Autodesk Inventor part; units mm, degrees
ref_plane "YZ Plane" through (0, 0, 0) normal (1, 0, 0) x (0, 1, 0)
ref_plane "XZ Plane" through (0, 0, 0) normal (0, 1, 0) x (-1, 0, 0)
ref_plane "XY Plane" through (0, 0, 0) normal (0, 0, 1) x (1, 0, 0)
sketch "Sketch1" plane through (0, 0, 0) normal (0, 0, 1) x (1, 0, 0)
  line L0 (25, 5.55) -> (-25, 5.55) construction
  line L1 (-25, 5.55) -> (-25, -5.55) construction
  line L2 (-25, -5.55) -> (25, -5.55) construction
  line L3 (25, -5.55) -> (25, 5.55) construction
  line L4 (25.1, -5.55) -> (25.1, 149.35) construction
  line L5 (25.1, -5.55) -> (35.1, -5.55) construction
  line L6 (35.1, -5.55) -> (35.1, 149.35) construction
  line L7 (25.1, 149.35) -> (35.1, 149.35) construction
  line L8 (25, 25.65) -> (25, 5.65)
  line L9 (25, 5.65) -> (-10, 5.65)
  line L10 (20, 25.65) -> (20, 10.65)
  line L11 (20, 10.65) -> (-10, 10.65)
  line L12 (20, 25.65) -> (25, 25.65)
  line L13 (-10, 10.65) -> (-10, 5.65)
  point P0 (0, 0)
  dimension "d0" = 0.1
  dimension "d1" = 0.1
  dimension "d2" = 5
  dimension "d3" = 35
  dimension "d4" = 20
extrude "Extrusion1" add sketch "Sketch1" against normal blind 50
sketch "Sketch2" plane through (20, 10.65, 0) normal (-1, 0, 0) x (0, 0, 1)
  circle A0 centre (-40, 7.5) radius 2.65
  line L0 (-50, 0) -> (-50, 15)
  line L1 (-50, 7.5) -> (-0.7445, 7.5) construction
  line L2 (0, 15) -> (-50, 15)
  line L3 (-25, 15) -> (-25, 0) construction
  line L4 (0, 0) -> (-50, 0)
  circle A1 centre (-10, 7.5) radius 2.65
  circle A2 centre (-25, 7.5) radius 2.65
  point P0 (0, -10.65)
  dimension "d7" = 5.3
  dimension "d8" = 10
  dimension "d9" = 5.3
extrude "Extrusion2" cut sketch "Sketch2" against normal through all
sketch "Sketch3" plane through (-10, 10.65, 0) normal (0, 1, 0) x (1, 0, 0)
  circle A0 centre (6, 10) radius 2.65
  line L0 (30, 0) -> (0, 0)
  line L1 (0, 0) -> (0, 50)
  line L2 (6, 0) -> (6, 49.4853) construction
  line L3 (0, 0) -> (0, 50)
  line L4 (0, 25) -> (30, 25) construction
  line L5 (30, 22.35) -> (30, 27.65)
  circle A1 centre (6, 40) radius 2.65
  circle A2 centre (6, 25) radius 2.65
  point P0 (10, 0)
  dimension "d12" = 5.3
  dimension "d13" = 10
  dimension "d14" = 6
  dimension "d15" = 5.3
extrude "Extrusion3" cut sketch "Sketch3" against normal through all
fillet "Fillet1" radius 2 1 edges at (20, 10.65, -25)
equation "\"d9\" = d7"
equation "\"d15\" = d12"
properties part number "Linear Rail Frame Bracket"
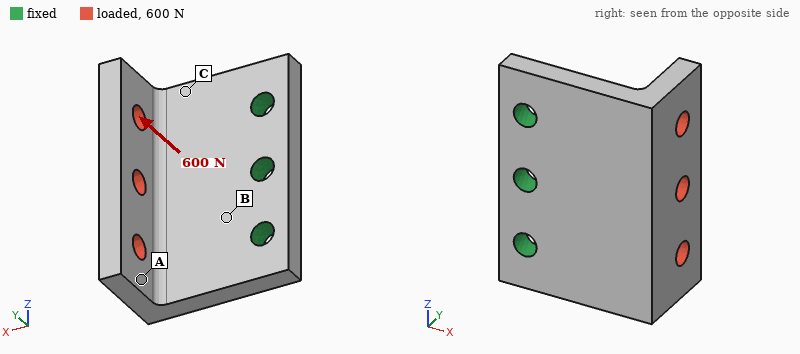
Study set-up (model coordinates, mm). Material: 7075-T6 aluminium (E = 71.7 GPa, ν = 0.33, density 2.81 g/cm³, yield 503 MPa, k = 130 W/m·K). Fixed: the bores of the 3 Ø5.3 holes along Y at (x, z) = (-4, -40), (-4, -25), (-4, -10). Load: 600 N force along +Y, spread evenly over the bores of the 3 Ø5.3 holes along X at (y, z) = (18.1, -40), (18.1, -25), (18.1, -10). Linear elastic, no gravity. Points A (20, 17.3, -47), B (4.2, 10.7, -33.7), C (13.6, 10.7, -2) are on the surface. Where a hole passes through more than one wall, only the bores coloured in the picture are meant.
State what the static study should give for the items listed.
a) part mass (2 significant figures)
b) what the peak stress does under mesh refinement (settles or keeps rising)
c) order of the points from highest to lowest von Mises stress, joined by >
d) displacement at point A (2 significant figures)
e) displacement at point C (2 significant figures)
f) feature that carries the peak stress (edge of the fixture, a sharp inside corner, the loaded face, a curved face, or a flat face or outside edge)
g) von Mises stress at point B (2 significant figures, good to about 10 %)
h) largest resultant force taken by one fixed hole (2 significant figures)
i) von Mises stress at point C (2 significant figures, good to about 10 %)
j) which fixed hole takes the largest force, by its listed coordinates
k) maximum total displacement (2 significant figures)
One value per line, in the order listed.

33 g
keeps rising
B > C > A
0.086 mm
0.044 mm
edge of the fixture
47 MPa
220 N
24 MPa
(-4, -25)
0.13 mm
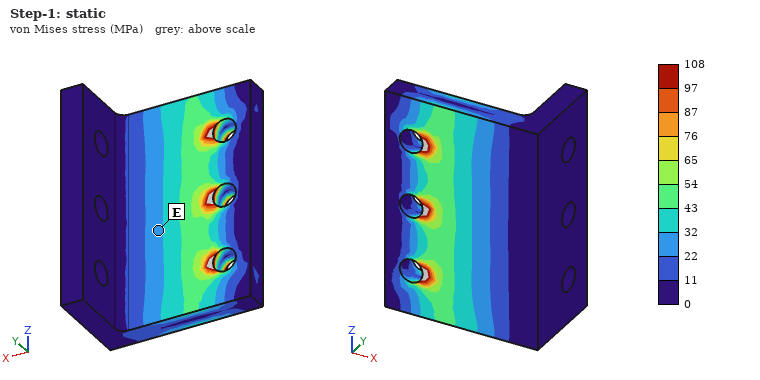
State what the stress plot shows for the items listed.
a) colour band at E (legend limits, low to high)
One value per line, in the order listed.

22 to 32 MPa
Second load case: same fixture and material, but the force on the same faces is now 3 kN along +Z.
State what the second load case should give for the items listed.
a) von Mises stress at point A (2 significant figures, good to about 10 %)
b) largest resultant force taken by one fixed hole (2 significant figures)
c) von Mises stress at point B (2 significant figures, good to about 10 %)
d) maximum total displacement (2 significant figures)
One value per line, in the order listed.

43 MPa
2.6 kN
86 MPa
0.21 mm
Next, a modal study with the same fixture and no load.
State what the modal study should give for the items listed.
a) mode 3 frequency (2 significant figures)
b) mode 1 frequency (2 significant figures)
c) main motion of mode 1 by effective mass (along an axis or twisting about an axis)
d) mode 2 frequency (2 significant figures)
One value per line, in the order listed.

10 kHz
3000 Hz
along Y
4900 Hz
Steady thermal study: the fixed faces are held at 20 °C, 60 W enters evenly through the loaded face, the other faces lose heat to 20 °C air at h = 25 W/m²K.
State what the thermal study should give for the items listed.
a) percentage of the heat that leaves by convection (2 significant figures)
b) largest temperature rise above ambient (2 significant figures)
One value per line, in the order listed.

7.2 %
65 K
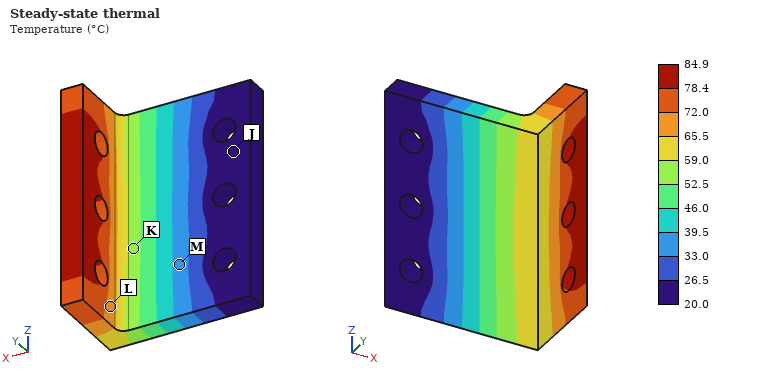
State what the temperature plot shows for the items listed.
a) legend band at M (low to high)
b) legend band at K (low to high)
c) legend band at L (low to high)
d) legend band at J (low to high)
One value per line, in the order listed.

33.0 to 39.5 °C
52.5 to 59.0 °C
65.5 to 72.0 °C
20.0 to 26.5 °C
